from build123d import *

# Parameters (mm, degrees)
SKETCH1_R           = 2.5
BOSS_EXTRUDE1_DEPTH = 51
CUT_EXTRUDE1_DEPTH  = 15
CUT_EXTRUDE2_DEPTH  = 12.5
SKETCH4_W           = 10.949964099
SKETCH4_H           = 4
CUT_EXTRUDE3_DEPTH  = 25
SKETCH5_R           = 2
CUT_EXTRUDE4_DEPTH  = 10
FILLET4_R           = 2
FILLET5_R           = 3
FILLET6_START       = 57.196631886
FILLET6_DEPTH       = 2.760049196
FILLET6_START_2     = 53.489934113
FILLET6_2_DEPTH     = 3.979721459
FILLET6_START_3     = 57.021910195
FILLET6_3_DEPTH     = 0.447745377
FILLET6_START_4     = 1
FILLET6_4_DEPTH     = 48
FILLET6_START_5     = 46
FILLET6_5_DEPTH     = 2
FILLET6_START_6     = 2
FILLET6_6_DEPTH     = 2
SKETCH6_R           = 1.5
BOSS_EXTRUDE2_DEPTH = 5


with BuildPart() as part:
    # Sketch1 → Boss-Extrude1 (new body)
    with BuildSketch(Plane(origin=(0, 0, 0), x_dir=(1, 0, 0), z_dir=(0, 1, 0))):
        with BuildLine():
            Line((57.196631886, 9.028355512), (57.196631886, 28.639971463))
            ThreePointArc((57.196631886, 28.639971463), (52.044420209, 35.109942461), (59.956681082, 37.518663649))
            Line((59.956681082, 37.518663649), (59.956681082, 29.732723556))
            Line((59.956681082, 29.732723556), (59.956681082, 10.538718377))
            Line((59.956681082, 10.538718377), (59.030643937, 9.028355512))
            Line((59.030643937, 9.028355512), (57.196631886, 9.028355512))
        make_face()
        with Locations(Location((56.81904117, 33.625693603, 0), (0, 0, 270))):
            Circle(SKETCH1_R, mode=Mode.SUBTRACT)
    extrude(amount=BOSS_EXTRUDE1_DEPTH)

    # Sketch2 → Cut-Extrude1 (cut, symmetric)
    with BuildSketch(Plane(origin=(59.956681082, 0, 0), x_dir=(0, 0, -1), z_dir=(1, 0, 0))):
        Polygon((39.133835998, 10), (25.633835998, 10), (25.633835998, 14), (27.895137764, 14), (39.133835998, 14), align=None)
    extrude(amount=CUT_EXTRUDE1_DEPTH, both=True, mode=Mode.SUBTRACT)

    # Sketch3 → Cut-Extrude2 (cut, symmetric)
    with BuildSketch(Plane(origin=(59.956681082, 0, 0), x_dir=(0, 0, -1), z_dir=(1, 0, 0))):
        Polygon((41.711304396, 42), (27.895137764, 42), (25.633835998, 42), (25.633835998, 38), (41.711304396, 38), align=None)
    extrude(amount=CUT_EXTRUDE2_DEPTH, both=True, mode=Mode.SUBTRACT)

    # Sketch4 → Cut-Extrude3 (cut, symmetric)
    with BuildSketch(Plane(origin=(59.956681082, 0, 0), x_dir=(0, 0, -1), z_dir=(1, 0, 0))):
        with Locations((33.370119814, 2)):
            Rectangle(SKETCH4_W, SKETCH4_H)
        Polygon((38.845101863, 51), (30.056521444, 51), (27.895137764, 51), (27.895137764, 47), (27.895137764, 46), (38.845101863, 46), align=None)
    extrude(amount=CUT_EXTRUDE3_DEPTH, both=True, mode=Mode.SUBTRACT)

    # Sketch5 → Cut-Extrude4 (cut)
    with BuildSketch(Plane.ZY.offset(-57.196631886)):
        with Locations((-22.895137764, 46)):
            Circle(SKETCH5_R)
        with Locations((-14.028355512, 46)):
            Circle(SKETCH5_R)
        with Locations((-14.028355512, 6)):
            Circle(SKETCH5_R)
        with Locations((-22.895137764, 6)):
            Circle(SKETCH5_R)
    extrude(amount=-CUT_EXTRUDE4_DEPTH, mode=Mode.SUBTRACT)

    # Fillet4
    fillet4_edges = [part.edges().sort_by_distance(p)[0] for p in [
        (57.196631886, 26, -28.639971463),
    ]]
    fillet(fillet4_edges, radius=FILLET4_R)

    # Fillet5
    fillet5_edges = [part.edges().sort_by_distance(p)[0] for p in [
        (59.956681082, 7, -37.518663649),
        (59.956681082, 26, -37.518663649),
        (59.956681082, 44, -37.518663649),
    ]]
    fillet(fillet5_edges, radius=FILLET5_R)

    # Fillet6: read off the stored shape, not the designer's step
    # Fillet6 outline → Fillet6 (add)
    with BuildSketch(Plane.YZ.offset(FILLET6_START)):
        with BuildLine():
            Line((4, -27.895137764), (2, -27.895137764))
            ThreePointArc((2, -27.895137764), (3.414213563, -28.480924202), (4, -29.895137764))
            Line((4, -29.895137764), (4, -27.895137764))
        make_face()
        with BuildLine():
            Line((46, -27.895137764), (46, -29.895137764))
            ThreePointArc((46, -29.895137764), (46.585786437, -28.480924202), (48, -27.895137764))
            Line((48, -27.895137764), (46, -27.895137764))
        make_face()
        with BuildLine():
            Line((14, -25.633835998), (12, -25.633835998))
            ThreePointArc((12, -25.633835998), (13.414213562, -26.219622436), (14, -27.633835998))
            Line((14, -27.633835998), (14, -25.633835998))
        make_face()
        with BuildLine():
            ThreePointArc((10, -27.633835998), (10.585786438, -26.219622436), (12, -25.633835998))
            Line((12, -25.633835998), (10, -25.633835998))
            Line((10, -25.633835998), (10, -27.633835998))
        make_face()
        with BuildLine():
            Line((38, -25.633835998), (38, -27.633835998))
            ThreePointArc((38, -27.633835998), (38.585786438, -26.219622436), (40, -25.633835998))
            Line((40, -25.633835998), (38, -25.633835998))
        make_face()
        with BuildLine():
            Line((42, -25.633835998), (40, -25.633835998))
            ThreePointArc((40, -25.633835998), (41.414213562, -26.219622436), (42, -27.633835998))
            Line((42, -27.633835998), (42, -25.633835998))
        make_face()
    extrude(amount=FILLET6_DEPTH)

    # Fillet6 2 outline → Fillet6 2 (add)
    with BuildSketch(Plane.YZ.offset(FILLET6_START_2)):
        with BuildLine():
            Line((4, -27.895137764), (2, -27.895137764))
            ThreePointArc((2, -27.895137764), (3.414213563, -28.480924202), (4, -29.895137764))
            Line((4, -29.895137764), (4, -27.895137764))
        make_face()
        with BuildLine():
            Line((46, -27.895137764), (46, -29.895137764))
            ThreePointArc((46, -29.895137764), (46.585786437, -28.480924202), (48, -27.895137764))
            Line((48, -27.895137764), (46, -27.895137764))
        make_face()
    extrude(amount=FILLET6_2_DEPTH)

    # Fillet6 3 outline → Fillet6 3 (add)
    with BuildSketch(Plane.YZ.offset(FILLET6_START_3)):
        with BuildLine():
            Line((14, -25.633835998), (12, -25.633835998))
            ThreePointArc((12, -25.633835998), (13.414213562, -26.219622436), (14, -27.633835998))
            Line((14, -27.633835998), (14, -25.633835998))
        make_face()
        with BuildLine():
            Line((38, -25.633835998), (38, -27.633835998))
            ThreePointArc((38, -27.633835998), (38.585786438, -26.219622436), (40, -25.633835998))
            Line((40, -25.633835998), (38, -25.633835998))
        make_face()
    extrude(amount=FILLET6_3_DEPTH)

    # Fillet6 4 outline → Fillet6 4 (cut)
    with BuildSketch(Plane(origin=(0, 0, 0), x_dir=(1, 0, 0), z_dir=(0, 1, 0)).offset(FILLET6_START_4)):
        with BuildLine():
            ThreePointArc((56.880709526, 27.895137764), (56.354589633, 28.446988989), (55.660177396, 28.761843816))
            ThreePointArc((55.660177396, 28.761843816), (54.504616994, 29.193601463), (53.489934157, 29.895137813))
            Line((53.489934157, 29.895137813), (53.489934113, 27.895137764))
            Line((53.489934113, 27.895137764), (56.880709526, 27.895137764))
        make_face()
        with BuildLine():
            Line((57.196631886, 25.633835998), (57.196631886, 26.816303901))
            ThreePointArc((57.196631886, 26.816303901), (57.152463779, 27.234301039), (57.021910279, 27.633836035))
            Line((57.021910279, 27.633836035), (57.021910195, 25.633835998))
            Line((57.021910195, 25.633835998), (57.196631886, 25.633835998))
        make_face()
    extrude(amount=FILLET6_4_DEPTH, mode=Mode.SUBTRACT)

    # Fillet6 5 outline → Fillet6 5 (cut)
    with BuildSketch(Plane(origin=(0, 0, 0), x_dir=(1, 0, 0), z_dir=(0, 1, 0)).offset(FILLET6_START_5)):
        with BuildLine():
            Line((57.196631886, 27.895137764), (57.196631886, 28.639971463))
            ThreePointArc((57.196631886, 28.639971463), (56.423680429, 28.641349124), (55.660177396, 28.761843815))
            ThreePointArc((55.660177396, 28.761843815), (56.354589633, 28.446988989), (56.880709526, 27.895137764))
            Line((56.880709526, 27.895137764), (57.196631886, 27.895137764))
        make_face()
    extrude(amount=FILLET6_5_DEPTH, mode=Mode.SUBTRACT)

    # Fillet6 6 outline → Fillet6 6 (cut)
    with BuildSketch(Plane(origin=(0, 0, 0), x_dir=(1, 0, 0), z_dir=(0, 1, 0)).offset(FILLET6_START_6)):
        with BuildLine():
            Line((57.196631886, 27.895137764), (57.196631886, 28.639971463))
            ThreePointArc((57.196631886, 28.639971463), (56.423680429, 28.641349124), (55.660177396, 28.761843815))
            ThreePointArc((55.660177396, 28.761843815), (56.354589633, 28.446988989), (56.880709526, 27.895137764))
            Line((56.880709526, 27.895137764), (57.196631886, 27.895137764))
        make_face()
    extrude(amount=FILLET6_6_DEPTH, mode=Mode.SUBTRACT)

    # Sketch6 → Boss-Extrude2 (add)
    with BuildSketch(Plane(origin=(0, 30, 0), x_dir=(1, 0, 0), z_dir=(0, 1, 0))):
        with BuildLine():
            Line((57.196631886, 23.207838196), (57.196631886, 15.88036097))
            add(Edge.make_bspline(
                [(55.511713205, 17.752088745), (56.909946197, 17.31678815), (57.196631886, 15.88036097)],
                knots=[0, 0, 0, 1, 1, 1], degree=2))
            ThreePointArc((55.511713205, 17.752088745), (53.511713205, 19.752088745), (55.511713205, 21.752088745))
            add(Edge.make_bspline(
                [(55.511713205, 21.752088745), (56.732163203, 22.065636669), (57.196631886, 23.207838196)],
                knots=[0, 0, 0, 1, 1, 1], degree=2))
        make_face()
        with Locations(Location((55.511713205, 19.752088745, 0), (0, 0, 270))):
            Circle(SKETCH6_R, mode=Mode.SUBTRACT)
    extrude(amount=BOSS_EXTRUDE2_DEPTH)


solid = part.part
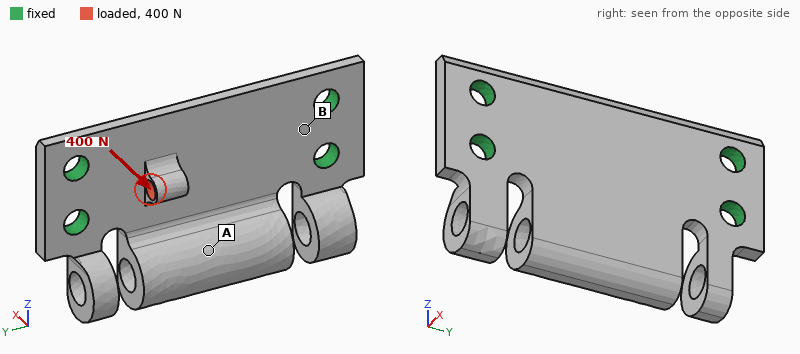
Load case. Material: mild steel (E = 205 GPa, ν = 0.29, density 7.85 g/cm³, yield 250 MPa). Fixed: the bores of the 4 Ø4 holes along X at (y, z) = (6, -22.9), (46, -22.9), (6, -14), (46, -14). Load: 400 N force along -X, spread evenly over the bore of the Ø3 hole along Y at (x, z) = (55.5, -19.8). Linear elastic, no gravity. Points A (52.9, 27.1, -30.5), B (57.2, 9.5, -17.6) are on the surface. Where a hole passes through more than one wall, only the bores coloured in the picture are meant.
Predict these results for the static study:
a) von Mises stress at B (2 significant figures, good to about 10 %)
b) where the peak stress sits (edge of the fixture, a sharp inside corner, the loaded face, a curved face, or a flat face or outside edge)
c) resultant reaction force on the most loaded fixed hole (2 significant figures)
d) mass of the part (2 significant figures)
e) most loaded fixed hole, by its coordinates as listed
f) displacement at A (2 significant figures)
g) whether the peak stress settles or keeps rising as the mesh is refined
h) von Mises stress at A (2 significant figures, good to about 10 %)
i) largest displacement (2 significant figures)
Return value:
22 MPa
edge of the fixture
180 N
33 g
(46, -22.9)
6.6 µm
keeps rising
9.2 MPa
11 µm
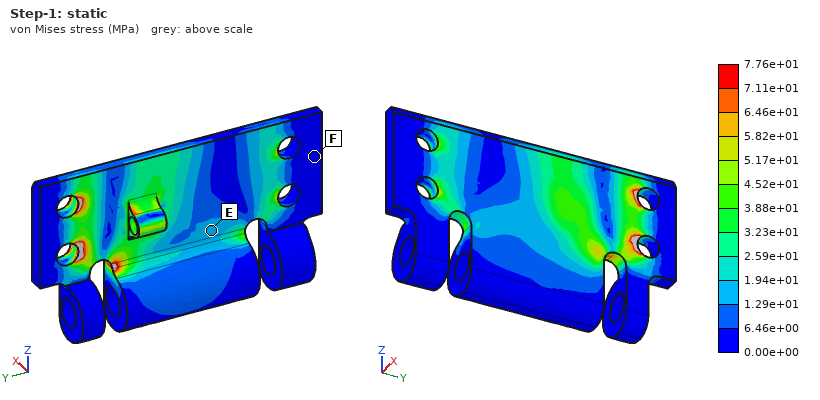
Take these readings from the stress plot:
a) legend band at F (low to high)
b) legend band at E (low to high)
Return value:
0.00e+00 to 6.46e+00 MPa
1.29e+01 to 1.94e+01 MPa
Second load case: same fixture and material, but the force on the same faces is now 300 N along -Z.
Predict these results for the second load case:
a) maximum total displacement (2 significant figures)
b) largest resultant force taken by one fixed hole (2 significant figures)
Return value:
7.2 µm
160 N
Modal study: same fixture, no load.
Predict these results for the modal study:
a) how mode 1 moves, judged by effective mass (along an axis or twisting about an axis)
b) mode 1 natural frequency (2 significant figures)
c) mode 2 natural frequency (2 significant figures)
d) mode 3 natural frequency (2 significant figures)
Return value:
along X
4100 Hz
8500 Hz
8800 Hz
